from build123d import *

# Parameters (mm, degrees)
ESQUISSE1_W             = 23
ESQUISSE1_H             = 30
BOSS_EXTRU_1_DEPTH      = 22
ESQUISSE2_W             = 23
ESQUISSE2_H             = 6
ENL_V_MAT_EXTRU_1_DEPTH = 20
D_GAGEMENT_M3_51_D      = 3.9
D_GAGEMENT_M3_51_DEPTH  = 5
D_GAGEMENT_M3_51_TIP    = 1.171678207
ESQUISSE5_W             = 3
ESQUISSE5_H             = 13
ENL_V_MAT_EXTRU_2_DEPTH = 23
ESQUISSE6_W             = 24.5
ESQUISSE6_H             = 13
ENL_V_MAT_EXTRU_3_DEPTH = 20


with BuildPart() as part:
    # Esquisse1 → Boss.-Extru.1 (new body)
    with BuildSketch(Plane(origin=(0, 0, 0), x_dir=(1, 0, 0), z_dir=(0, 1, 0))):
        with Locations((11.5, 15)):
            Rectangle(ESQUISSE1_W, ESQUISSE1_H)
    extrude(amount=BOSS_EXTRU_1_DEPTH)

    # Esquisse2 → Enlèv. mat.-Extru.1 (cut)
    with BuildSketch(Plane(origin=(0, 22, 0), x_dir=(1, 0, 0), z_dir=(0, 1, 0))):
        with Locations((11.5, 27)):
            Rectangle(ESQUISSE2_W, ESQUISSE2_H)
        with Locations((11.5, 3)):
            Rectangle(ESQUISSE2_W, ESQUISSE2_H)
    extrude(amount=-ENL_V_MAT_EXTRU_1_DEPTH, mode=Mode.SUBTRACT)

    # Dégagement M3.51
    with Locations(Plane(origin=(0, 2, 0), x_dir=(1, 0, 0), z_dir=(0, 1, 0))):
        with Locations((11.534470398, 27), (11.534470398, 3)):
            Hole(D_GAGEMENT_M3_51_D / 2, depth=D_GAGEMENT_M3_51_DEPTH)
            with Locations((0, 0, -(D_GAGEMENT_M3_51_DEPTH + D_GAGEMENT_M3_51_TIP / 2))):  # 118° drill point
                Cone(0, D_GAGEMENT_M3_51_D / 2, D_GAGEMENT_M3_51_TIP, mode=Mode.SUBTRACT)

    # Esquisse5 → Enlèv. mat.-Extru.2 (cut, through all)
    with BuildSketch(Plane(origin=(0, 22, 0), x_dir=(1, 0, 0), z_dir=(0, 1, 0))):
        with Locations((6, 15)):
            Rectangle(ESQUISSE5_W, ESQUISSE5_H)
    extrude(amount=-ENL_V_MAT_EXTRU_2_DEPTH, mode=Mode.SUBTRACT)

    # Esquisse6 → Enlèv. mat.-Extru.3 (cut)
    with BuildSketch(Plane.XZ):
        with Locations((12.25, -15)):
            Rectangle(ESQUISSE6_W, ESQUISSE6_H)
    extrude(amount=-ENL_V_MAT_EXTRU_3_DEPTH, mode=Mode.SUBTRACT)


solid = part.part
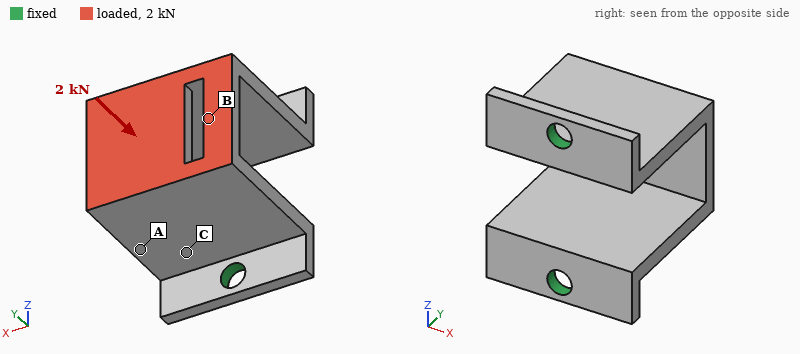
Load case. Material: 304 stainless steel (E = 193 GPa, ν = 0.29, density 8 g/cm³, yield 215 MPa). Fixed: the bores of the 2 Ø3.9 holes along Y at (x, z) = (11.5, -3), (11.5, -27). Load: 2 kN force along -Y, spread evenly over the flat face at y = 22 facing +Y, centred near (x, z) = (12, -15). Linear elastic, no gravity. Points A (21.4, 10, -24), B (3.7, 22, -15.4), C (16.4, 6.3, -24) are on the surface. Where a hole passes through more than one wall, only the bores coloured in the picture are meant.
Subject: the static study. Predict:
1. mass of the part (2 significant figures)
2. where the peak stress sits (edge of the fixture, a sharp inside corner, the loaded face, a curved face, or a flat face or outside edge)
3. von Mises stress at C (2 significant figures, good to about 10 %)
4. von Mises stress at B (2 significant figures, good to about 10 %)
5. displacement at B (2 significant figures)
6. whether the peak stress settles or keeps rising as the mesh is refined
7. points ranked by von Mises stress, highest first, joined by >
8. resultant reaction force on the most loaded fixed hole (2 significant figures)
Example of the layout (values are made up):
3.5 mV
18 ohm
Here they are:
28 g
edge of the fixture
52 MPa
97 MPa
15 µm
keeps rising
B > C > A
1.0 kN
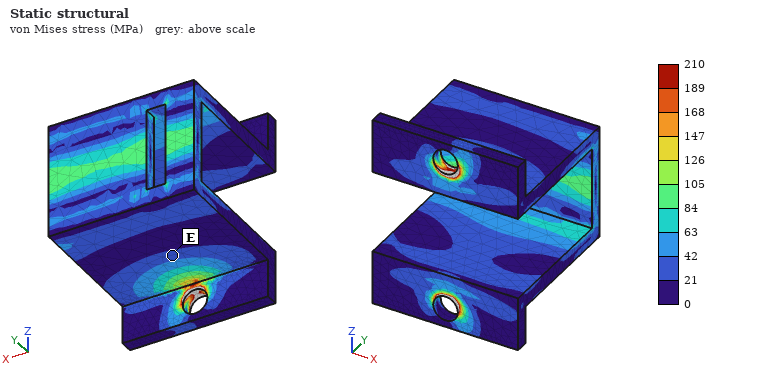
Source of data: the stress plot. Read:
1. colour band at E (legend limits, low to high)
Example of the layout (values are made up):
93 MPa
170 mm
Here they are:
21 to 42 MPa
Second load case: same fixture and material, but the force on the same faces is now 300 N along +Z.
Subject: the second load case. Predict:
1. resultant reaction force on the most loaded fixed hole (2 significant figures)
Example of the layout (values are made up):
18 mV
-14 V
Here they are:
270 N
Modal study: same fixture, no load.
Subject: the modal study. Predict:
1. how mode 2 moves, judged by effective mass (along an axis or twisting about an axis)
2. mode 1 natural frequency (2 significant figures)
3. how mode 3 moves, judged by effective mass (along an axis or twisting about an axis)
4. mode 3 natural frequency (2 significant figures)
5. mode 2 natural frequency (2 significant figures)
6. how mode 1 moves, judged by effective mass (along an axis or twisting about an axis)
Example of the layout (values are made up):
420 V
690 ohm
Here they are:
along Z
3600 Hz
twisting about Y
6100 Hz
4000 Hz
along X
